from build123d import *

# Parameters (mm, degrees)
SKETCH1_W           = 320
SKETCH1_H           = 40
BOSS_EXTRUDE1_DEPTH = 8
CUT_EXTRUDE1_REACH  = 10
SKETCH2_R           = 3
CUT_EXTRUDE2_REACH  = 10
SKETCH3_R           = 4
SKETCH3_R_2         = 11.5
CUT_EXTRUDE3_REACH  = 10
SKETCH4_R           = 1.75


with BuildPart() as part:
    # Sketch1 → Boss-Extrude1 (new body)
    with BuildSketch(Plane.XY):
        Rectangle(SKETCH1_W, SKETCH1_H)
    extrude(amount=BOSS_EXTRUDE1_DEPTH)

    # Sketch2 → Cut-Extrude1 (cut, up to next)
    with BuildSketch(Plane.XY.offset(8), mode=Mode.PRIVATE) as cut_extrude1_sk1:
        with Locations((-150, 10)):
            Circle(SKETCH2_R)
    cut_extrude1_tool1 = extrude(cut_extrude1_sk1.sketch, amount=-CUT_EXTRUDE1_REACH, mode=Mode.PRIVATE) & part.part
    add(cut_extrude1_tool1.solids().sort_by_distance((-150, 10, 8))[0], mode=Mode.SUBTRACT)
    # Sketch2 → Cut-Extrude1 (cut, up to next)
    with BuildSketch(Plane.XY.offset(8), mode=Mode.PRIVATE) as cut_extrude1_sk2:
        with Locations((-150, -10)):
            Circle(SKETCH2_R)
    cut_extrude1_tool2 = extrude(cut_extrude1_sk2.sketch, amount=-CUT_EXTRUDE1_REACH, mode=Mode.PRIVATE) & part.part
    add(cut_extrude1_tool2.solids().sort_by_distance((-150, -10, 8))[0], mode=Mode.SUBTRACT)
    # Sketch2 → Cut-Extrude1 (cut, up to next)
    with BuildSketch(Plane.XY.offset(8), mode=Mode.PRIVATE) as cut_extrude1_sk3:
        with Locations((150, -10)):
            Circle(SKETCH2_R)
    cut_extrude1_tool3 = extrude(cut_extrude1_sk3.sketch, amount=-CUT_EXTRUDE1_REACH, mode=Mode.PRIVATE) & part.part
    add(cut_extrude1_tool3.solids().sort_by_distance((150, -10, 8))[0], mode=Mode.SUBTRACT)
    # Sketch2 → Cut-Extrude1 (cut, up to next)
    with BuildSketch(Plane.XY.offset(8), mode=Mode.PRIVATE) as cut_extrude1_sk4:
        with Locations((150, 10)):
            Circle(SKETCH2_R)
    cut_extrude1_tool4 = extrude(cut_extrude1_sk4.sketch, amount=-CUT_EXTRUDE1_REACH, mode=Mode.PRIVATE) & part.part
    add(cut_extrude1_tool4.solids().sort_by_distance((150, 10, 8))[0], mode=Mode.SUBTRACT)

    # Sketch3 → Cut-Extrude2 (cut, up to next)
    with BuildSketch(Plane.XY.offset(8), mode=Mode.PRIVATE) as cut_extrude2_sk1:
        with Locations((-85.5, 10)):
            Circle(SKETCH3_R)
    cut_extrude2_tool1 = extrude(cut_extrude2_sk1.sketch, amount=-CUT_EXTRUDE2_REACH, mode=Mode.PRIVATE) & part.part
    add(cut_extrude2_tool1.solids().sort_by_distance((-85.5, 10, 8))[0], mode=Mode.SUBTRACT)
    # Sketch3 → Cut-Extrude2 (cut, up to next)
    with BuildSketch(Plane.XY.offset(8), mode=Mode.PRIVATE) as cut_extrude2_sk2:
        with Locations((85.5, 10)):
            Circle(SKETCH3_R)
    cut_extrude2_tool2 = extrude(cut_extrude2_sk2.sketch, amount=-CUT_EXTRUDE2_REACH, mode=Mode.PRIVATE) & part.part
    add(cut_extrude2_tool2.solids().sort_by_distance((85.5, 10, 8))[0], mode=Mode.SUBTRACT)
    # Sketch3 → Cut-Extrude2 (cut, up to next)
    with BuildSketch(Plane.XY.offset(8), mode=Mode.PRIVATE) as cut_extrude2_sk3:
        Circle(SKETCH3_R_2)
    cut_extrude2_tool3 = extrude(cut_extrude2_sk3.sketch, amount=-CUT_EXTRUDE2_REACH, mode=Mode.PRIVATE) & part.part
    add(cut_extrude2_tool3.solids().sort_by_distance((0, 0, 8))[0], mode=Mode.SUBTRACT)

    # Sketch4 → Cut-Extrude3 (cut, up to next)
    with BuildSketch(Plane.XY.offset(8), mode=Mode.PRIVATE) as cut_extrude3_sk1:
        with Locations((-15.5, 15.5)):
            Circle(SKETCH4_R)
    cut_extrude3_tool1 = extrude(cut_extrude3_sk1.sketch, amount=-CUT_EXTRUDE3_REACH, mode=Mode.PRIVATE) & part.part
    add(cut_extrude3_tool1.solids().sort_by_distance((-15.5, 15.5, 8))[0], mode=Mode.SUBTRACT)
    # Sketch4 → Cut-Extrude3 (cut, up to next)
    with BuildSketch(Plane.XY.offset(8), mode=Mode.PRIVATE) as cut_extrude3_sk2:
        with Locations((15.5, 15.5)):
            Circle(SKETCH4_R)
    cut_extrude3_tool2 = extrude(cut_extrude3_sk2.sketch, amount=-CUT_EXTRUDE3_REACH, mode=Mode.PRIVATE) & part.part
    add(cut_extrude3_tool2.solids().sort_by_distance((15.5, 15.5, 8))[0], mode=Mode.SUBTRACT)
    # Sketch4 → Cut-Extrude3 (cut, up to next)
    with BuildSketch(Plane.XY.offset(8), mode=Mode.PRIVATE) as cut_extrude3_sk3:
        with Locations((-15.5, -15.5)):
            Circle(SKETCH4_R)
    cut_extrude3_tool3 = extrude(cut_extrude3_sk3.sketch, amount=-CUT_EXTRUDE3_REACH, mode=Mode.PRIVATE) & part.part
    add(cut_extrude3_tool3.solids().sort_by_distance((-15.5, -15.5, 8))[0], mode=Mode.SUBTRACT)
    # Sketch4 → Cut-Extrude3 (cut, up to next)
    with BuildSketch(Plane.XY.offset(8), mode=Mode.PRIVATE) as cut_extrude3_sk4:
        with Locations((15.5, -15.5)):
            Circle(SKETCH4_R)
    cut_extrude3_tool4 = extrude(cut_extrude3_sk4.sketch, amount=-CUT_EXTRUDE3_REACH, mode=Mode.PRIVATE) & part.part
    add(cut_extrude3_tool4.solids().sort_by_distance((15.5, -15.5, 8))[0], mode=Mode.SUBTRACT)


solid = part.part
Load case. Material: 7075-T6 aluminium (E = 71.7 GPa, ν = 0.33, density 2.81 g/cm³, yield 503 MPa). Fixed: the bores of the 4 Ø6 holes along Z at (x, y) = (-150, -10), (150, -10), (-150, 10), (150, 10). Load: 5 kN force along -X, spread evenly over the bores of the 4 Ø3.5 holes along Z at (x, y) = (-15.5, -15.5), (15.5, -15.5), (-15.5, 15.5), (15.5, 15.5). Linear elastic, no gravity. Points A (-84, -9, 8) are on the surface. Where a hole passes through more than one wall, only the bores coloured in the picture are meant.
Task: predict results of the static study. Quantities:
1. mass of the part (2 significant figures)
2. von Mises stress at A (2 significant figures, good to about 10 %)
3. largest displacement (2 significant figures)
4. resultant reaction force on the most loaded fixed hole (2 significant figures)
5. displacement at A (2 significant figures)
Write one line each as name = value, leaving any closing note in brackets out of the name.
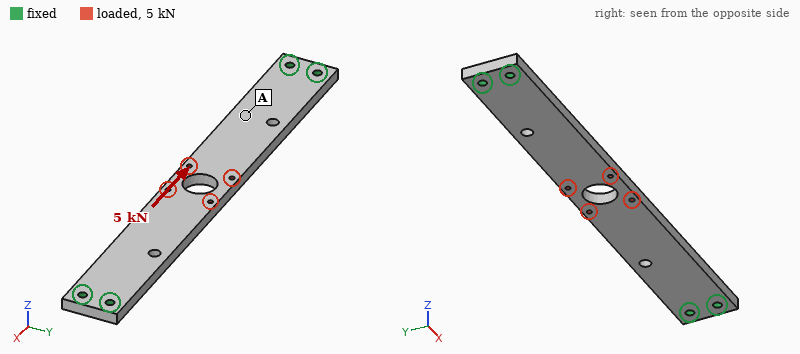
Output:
mass of the part = 270 g
von Mises stress at A = 7.9 MPa
largest displacement = 17 µm
resultant reaction force on the most loaded fixed hole = 1.3 kN
displacement at A = 7.6 µm
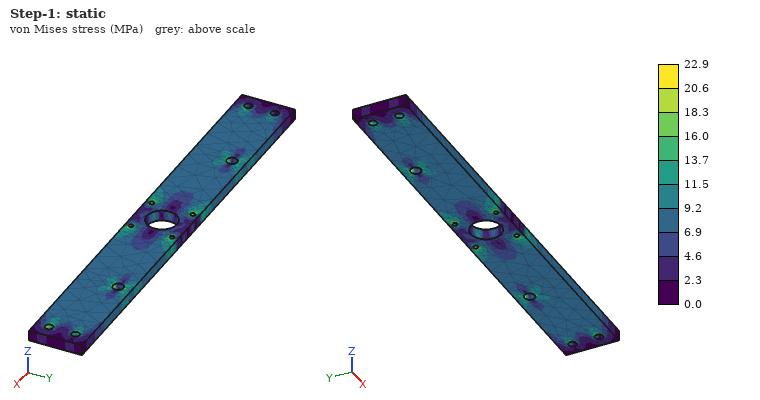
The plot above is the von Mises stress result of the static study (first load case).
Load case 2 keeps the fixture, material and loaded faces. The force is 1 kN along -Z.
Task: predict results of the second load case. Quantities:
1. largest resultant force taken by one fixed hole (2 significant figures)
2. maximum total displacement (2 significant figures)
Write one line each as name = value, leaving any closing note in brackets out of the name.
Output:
largest resultant force taken by one fixed hole = 250 N
maximum total displacement = 1.4 mm
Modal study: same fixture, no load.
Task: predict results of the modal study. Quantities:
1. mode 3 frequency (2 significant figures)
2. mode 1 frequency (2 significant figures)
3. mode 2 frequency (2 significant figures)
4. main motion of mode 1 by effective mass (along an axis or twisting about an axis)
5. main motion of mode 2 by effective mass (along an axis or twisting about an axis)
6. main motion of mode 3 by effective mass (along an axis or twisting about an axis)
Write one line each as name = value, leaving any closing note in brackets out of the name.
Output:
mode 3 frequency = 2000 Hz
mode 1 frequency = 460 Hz
mode 2 frequency = 1300 Hz
main motion of mode 1 by effective mass = along Z
main motion of mode 2 by effective mass = twisting about Y
main motion of mode 3 by effective mass = twisting about X
